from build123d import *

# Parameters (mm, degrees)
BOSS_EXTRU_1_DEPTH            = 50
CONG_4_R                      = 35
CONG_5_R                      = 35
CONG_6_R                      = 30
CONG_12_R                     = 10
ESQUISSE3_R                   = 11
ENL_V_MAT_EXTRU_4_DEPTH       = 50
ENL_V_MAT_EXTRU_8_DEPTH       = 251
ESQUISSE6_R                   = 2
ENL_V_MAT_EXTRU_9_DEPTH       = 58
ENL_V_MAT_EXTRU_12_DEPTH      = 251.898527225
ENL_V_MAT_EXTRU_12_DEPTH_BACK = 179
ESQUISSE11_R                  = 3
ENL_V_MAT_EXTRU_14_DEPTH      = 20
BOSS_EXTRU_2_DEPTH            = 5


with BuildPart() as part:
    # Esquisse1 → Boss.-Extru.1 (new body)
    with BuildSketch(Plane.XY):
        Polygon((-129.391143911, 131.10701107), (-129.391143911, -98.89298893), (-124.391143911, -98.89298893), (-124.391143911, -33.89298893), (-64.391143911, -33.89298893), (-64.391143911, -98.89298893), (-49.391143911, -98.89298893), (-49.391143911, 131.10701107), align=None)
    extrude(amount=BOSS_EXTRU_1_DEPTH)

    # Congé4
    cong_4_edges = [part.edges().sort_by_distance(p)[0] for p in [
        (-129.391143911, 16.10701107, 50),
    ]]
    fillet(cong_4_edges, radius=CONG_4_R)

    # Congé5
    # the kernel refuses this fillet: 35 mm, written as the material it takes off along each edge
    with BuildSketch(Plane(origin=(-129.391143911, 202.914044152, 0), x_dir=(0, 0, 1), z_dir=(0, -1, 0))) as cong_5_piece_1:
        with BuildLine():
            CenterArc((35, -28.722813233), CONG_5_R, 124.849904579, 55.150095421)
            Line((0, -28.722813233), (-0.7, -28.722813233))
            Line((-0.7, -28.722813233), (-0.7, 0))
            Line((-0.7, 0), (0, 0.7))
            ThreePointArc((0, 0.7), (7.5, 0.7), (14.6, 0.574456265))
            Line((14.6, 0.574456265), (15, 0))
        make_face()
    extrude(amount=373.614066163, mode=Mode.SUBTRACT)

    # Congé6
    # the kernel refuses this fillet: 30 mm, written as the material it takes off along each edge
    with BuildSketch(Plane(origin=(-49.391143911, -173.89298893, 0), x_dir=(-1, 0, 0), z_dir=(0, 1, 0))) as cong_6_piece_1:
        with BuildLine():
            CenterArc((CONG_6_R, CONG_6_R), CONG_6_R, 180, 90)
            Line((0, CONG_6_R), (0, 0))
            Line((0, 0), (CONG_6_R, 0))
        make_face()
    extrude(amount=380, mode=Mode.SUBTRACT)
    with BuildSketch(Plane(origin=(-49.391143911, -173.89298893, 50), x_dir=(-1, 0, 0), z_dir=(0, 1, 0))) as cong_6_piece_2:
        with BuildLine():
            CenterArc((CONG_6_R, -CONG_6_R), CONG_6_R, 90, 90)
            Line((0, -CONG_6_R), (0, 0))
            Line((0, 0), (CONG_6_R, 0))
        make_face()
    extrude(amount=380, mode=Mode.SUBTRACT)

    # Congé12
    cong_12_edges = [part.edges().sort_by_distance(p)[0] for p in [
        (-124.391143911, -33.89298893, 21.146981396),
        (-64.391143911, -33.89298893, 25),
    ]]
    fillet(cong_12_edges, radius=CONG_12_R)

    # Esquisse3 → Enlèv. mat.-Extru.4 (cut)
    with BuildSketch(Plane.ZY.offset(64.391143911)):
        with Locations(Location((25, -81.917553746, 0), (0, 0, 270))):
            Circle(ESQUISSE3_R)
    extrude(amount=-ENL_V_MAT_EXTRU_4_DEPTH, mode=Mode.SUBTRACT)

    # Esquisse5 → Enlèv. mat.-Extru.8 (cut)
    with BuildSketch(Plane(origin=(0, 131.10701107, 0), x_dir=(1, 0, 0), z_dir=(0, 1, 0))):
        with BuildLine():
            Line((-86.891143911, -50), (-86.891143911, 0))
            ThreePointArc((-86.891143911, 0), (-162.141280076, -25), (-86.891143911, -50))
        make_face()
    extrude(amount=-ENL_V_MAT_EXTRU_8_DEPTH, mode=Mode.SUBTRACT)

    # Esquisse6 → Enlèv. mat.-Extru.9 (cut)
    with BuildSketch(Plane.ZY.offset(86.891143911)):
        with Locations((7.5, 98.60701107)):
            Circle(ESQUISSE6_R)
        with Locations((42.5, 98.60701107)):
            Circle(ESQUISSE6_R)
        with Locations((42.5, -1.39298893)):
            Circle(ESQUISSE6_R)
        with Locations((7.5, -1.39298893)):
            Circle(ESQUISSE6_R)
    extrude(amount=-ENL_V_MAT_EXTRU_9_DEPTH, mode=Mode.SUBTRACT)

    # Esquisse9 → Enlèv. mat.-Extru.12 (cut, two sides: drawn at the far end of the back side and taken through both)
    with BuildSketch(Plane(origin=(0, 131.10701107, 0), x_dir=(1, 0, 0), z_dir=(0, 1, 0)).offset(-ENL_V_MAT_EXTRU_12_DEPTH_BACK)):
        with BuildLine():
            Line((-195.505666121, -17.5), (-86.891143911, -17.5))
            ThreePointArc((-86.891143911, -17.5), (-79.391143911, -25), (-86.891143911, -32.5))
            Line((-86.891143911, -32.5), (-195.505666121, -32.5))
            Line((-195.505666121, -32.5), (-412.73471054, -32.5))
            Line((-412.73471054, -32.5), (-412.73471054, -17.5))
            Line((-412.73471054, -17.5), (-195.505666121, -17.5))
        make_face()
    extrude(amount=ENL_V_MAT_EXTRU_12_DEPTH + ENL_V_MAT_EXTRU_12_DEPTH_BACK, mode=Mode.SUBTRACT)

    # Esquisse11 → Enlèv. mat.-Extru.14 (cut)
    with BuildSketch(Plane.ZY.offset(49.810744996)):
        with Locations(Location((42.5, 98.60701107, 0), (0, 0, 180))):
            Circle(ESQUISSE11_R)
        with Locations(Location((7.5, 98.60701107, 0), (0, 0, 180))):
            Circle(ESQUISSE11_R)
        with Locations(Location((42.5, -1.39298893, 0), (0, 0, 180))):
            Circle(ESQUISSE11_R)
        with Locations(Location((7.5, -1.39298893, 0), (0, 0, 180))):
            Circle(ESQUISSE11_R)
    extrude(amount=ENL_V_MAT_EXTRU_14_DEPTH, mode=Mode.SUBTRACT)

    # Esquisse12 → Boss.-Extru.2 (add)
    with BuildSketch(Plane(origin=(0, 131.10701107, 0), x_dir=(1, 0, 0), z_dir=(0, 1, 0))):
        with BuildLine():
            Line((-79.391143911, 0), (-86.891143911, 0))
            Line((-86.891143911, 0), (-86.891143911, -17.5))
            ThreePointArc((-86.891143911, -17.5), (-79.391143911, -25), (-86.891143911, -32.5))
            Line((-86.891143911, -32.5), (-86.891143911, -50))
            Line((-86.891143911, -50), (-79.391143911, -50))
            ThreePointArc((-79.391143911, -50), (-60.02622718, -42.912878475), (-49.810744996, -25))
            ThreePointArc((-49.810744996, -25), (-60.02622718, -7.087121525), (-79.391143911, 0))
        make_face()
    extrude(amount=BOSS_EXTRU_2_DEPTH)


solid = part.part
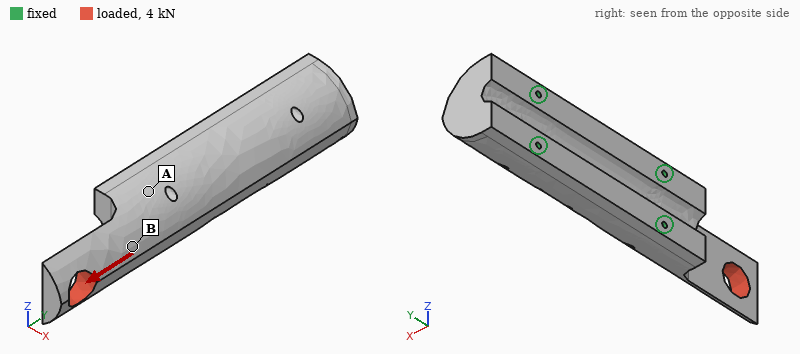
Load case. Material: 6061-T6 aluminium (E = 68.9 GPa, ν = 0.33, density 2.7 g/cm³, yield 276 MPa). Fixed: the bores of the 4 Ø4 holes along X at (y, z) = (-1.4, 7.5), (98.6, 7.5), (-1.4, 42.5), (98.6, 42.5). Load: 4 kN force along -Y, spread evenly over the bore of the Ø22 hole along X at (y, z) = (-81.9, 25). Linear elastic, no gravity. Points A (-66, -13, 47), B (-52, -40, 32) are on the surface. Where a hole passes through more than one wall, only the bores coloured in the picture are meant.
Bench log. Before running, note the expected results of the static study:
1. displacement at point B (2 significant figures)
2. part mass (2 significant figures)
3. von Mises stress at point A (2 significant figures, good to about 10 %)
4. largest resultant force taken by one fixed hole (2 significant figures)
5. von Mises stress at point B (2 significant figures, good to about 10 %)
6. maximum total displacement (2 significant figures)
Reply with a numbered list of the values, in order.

1. 17 µm
2. 700 g
3. 5.9 MPa
4. 1.3 kN
5. 13 MPa
6. 90 µm
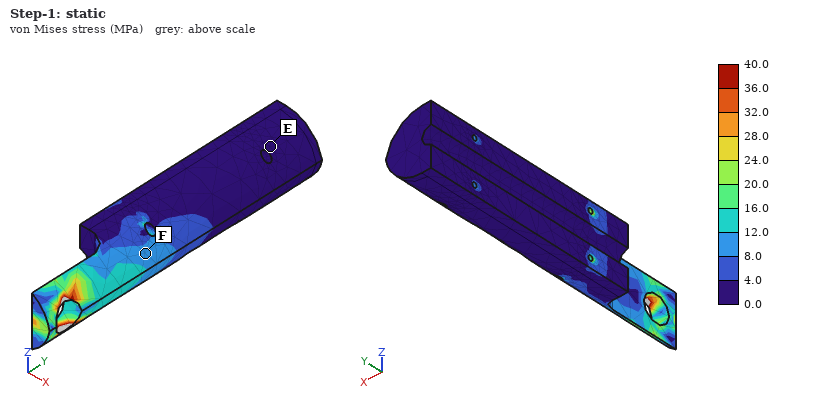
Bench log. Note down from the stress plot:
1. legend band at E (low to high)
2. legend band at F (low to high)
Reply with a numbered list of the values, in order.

1. 0.0 to 4.0 MPa
2. 8.0 to 12.0 MPa
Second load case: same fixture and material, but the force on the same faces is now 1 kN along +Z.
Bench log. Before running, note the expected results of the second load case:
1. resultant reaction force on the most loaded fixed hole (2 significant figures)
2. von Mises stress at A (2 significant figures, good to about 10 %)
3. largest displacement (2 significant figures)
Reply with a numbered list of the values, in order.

1. 2.0 kN
2. 8.3 MPa
3. 66 µm
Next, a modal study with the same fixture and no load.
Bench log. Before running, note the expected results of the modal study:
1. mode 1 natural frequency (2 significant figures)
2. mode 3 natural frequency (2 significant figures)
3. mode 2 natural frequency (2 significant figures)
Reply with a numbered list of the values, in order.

1. 2300 Hz
2. 6400 Hz
3. 4200 Hz
